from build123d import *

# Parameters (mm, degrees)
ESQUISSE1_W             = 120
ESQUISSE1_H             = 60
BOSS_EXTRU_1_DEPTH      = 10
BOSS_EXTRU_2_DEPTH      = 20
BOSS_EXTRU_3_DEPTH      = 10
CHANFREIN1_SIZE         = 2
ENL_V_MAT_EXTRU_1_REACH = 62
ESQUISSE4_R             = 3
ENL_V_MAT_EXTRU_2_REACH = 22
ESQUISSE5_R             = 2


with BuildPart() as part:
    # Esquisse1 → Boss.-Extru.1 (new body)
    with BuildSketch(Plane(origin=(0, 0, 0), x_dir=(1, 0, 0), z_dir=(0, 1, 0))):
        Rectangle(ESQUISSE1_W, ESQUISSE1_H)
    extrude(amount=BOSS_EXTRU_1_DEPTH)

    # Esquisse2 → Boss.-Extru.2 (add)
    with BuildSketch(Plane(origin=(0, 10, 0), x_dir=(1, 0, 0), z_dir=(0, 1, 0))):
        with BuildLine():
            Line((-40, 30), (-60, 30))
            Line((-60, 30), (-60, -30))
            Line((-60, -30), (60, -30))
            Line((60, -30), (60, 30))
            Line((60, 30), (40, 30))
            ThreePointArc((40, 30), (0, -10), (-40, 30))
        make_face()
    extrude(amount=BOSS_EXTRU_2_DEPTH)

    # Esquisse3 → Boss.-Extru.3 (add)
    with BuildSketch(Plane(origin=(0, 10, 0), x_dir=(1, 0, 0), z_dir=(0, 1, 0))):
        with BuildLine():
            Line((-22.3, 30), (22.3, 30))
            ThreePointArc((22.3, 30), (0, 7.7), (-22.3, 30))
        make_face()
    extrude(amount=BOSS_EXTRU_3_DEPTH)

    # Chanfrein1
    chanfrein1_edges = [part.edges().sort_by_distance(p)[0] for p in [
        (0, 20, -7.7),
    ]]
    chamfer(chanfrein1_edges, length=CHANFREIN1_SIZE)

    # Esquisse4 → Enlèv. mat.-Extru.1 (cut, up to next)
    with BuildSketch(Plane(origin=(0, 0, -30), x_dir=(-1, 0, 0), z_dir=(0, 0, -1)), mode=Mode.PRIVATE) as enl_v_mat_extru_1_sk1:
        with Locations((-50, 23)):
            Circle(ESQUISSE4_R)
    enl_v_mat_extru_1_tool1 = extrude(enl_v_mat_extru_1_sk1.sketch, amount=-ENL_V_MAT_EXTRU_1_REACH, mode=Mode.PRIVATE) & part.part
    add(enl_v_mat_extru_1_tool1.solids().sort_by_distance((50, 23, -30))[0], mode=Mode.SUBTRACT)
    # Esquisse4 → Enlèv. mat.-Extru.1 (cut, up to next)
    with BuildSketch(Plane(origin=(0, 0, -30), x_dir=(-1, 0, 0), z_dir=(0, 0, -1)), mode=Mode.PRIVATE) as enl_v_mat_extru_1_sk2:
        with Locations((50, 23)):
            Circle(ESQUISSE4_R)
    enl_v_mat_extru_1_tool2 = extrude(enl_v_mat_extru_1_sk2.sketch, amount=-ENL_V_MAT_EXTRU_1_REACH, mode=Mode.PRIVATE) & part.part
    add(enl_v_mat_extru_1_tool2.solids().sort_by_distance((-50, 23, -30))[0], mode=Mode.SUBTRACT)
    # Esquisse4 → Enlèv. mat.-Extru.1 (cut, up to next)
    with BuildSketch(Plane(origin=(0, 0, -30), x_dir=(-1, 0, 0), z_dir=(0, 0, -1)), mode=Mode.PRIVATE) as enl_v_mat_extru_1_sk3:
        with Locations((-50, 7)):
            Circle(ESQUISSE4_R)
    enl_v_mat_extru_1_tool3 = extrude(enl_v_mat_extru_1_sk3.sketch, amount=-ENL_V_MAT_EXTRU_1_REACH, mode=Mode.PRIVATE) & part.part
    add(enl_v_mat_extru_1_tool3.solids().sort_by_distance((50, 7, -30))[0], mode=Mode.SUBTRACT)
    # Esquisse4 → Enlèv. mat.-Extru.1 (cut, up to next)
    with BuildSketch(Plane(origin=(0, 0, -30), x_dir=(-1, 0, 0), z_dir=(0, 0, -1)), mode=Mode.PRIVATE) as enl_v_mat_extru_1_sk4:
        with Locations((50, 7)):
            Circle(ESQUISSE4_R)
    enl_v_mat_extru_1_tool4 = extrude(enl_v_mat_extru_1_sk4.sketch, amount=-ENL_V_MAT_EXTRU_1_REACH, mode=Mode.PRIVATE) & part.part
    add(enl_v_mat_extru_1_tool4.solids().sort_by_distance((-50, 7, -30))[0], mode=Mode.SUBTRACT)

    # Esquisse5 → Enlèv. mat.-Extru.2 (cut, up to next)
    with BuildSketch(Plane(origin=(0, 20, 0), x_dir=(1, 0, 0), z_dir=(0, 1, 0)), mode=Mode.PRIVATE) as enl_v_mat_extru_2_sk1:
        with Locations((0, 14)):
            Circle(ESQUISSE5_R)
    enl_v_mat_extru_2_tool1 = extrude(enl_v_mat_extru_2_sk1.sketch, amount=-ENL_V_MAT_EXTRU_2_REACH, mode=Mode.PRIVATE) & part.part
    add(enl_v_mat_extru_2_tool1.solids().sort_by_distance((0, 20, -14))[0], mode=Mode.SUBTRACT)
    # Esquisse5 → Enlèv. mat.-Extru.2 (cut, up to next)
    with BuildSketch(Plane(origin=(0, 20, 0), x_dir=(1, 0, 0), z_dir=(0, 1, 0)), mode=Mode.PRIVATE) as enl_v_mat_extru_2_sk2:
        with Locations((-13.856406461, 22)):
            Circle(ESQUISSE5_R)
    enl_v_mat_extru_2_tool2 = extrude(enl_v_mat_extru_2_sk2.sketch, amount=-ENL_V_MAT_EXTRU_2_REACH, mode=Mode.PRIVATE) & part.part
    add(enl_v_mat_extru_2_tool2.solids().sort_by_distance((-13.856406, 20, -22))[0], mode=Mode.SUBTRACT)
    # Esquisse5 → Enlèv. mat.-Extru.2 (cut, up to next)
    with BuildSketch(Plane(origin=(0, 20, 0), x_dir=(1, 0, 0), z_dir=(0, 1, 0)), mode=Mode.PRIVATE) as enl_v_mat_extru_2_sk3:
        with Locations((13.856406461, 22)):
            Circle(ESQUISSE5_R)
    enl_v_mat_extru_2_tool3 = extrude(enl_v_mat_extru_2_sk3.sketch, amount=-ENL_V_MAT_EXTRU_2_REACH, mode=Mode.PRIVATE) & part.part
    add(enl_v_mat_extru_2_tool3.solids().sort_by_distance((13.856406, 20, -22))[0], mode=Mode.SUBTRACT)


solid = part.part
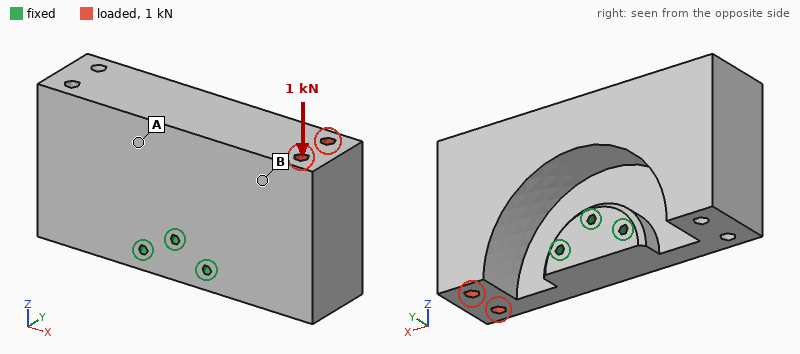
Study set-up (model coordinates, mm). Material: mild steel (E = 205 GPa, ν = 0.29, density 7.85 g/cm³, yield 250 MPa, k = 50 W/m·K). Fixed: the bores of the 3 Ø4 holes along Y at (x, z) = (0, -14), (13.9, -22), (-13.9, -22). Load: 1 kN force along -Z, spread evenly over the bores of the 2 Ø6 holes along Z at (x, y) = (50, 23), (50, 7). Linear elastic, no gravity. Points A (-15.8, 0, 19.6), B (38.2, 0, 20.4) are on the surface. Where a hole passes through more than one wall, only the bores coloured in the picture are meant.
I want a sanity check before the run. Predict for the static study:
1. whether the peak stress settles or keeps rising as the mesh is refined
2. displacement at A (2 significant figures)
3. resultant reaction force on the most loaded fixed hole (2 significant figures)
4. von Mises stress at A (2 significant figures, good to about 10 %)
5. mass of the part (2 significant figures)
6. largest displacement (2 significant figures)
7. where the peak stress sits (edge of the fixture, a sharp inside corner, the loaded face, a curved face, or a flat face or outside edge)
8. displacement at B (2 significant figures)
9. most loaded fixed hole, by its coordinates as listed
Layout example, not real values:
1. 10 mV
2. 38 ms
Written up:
1. keeps rising
2. 3.1 µm
3. 1.9 kN
4. 3.0 MPa
5. 1.3 kg
6. 8.9 µm
7. edge of the fixture
8. 5.0 µm
9. (13.9, -22)
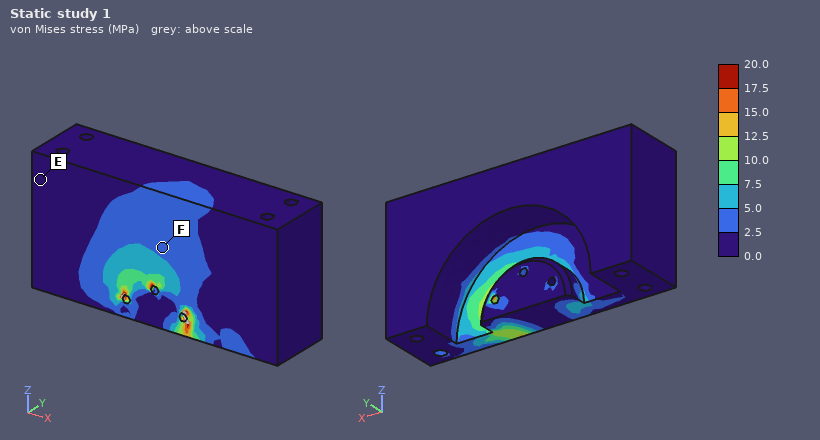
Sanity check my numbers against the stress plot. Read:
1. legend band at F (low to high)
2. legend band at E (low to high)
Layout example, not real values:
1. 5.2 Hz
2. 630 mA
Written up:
1. 2.5 to 5.0 MPa
2. 0.0 to 2.5 MPa
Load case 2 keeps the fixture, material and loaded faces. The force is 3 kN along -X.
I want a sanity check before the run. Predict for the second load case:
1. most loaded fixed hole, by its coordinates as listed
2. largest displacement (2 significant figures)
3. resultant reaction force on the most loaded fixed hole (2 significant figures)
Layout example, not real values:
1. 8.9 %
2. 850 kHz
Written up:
1. (0, -14)
2. 14 µm
3. 2.1 kN
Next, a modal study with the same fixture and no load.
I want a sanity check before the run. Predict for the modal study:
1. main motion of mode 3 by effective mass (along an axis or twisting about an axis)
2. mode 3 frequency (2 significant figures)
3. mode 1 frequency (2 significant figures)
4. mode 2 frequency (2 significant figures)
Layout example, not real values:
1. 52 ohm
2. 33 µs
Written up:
1. along X
2. 2900 Hz
3. 1800 Hz
4. 1800 Hz
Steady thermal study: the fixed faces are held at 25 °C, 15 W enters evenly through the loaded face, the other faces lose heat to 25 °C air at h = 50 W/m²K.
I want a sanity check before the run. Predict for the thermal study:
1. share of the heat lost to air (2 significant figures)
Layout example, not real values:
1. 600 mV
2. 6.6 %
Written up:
1. 46 %
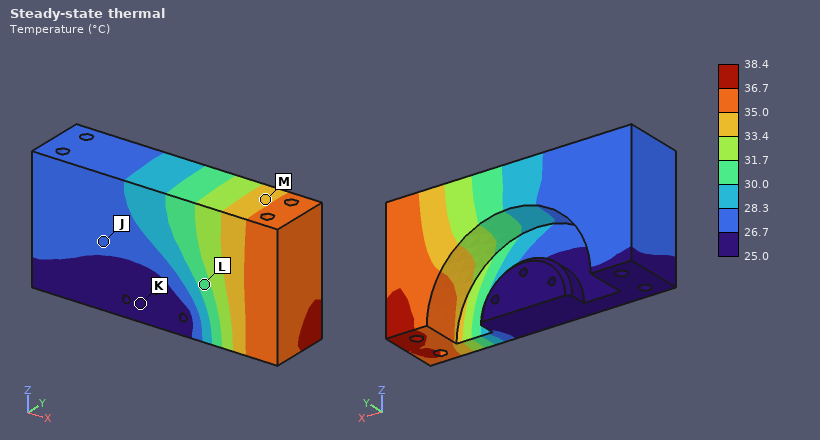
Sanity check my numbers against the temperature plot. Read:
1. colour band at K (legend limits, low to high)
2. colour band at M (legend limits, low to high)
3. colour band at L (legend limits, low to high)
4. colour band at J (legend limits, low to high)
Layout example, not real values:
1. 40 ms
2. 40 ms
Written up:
1. 25.0 to 26.7 °C
2. 33.4 to 35.0 °C
3. 30.0 to 31.7 °C
4. 26.7 to 28.3 °C
